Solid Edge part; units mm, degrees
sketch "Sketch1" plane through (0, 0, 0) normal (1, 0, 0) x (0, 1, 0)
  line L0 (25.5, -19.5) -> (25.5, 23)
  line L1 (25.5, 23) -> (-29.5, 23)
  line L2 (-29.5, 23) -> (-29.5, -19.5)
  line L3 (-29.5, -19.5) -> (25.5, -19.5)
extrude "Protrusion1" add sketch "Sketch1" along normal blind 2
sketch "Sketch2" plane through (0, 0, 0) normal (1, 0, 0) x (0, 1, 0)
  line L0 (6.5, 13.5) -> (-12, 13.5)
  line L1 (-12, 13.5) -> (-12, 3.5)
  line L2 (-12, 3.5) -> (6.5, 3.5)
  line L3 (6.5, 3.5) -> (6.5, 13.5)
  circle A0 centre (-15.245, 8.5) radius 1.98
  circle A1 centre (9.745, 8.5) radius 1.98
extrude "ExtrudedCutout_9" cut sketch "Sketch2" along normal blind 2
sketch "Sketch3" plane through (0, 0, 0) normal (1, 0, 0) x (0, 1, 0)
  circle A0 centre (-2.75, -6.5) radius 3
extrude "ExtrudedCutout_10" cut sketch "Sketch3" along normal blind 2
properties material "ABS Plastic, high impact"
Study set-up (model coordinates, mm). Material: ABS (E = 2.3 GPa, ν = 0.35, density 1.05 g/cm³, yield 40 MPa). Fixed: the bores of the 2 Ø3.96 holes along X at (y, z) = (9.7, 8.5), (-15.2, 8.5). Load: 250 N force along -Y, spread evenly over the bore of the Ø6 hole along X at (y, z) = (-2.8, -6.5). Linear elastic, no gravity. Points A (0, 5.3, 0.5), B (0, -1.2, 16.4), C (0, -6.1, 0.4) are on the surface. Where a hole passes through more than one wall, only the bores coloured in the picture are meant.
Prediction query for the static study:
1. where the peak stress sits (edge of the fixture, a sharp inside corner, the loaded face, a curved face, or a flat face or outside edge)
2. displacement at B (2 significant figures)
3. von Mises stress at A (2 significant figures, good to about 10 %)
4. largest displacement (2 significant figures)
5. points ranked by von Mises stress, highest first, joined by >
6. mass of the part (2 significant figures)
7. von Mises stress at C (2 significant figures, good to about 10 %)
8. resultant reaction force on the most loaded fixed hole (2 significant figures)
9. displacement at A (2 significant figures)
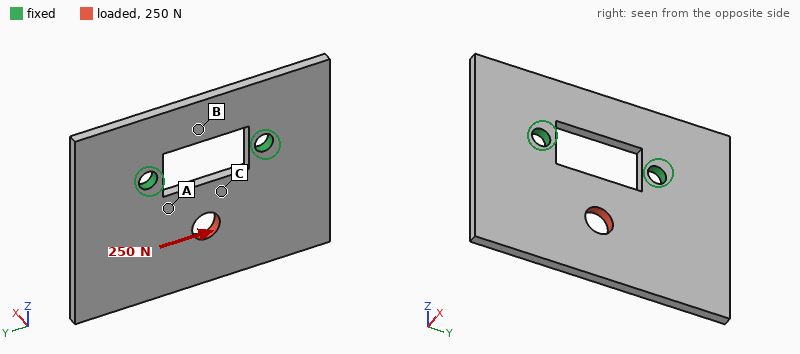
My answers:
edge of the fixture
0.033 mm
8.9 MPa
0.20 mm
A > C > B
4.4 g
6.4 MPa
170 N
0.084 mm
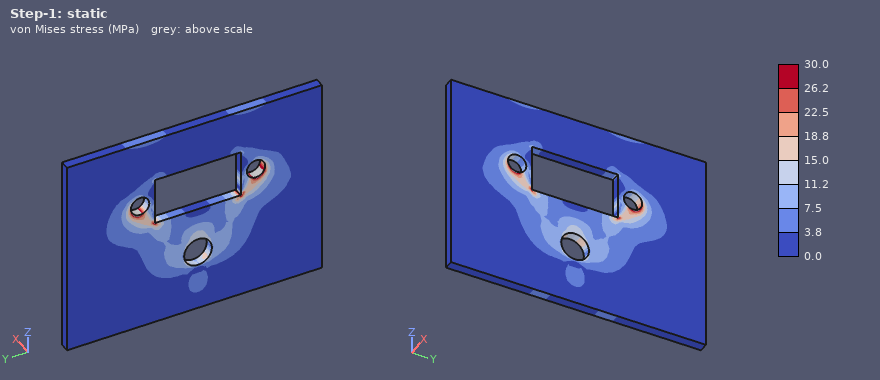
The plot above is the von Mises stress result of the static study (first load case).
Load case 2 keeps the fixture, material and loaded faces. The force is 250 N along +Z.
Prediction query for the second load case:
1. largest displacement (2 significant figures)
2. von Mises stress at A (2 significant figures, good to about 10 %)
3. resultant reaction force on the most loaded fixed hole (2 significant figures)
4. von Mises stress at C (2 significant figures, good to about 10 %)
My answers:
84 µm
8.8 MPa
130 N
5.0 MPa
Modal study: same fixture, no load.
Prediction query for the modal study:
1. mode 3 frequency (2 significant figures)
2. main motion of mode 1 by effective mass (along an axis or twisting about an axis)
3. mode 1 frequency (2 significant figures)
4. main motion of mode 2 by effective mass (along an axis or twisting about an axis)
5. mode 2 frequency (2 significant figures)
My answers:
1400 Hz
along X
520 Hz
twisting about Z
820 Hz
